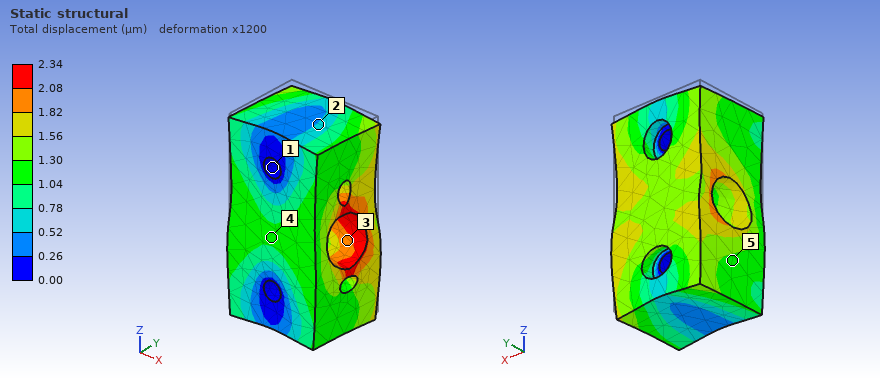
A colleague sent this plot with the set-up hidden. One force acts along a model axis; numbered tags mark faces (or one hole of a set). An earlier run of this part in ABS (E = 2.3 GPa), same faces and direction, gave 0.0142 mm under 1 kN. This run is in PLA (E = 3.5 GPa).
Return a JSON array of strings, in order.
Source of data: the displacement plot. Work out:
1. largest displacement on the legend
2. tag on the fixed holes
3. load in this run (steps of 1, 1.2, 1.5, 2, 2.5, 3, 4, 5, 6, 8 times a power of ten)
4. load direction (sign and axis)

["2.34 µm", "1", "250 N", "-Z"]
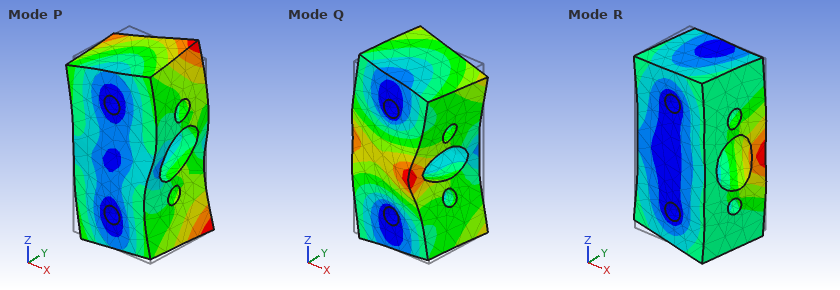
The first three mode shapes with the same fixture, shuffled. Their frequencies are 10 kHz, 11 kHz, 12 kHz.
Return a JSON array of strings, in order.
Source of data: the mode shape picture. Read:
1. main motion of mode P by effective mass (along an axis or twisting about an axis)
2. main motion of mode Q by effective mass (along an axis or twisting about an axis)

["twisting about Y", "twisting about Z"]
